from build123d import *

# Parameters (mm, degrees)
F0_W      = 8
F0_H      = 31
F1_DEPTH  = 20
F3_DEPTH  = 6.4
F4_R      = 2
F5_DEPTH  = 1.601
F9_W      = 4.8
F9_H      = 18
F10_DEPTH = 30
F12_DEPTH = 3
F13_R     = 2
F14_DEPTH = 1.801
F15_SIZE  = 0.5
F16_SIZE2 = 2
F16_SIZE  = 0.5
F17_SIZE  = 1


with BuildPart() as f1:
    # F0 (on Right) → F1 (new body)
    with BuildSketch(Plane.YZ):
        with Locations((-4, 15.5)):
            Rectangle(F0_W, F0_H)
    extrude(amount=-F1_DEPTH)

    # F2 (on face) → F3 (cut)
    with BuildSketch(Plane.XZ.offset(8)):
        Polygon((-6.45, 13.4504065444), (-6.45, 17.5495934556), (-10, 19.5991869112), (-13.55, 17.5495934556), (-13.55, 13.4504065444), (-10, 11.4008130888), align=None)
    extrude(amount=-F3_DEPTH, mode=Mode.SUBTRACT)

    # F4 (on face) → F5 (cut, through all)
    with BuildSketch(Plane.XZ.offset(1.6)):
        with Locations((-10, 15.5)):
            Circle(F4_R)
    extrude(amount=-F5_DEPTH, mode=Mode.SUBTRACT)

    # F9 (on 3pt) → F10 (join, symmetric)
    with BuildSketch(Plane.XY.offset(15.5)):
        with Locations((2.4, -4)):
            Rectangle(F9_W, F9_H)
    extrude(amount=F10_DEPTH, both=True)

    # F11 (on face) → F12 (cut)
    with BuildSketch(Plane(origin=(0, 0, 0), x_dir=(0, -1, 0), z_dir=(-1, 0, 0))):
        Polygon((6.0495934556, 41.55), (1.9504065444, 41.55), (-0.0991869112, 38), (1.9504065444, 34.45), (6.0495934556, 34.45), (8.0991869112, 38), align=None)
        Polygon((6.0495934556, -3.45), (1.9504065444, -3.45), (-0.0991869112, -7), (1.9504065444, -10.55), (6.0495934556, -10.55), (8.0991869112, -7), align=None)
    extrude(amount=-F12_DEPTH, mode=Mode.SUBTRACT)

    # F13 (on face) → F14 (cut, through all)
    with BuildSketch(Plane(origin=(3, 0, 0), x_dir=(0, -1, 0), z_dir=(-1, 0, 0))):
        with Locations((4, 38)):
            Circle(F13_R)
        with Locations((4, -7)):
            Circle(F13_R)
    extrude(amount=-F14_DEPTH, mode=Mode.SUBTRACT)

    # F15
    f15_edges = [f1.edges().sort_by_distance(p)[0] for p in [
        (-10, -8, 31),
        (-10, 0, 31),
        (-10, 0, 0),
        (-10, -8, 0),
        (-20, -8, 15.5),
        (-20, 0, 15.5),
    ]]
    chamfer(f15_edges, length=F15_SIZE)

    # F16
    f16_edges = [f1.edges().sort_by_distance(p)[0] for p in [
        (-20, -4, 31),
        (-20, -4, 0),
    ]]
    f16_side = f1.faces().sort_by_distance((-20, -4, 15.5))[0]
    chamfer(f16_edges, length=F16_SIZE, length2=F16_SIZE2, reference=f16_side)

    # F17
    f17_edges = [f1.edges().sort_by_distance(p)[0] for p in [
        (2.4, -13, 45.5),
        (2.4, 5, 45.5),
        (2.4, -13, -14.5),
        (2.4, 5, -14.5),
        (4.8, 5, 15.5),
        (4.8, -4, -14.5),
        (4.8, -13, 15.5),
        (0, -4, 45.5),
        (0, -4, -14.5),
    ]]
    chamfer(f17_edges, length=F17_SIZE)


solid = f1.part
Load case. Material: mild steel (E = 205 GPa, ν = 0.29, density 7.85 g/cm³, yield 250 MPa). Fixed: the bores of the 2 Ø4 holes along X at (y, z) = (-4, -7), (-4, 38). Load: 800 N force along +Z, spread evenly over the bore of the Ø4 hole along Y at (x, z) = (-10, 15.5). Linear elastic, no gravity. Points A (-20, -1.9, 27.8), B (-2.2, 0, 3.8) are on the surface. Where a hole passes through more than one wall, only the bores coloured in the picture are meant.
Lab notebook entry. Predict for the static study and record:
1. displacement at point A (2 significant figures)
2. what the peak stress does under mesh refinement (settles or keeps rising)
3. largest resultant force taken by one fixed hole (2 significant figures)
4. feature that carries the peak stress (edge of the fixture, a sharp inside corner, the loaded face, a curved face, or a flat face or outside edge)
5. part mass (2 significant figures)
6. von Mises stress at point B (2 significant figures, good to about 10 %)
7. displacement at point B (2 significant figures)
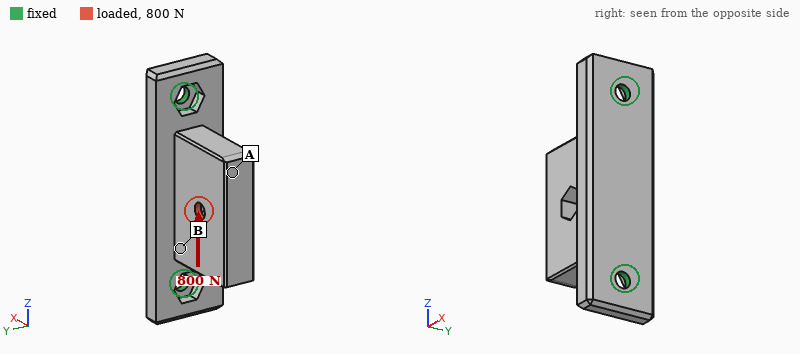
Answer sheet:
3.6 µm
keeps rising
480 N
edge of the fixture
74 g
15 MPa
1.3 µm
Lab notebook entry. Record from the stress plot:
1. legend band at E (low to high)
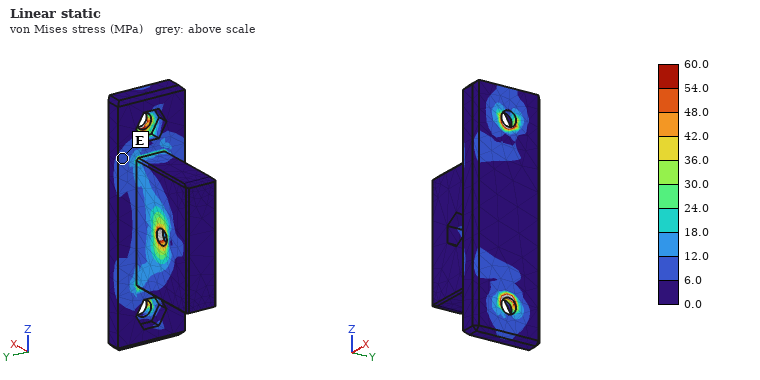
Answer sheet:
6.0 to 12.0 MPa
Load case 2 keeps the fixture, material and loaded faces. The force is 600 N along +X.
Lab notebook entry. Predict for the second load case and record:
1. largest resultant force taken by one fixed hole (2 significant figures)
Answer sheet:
420 N
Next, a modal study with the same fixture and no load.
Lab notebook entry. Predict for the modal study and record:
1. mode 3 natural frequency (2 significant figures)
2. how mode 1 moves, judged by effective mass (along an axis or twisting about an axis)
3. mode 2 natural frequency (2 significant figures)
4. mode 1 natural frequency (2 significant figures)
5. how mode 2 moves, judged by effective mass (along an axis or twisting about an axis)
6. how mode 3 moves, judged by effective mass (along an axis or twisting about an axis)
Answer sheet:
13 kHz
along Y
9700 Hz
3100 Hz
along X
along Z
